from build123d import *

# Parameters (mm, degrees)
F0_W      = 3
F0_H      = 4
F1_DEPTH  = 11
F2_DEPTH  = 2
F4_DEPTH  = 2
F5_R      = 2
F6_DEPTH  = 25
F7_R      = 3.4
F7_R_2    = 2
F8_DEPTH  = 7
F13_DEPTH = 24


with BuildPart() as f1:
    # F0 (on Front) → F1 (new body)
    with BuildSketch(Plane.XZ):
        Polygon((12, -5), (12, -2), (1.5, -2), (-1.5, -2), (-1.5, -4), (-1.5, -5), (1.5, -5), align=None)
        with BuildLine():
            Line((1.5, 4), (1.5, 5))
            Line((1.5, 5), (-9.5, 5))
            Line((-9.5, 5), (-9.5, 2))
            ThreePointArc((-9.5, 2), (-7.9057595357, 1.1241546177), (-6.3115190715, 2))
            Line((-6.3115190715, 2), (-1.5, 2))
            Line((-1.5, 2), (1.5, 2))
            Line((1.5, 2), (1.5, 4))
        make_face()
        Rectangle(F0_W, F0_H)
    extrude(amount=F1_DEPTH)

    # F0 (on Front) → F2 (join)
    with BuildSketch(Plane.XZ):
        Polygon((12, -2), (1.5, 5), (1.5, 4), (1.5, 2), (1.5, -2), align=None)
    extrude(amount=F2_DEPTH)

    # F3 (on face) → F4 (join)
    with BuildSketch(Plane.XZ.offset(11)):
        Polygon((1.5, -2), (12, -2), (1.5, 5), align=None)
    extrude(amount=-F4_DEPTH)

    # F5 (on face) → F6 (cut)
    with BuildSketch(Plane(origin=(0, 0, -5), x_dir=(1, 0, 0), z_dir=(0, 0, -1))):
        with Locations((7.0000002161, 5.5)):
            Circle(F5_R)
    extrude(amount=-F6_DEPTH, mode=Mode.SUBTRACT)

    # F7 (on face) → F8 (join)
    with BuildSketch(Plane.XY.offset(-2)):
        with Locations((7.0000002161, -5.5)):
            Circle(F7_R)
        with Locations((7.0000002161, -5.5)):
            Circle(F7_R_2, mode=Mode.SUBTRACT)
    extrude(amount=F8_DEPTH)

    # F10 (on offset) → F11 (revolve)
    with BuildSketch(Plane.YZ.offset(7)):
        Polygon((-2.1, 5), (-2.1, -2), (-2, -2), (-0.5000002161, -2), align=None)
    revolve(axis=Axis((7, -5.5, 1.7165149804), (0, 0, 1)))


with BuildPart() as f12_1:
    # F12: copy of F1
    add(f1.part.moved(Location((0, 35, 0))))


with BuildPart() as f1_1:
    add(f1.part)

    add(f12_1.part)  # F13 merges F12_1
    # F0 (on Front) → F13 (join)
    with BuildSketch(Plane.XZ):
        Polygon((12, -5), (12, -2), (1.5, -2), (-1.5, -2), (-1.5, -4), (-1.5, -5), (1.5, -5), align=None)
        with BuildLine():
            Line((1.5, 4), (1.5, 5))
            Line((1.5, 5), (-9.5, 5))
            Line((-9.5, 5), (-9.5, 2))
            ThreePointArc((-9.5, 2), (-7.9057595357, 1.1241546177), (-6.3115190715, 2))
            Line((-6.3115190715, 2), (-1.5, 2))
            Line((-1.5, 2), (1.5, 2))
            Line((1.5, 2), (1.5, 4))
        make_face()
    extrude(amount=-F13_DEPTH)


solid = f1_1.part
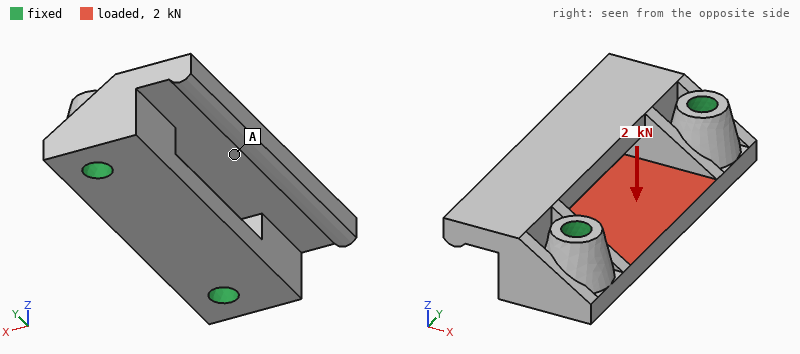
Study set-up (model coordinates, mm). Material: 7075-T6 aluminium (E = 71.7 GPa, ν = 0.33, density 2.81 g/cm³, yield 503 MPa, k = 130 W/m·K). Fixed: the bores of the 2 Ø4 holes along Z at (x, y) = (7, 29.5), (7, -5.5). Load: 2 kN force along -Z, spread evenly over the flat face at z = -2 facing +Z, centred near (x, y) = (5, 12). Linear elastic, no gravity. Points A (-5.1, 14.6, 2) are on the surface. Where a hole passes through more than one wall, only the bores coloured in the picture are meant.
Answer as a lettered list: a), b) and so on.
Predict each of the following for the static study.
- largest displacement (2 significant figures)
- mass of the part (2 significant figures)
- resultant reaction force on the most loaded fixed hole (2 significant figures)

a) 69 µm
b) 13 g
c) 1.0 kN
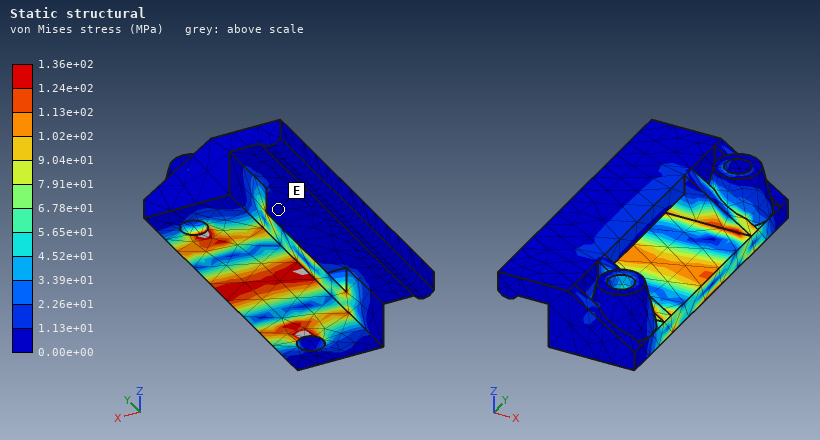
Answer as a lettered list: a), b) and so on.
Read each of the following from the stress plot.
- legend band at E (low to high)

a) 0.00e+00 to 1.13e+01 MPa
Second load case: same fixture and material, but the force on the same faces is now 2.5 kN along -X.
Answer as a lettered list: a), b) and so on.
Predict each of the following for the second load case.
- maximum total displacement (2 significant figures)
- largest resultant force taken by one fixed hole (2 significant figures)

a) 36 µm
b) 1.3 kN
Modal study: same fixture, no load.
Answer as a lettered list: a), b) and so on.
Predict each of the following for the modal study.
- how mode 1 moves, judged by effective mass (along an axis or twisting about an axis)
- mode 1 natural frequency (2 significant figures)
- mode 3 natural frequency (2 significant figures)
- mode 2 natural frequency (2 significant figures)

a) along Z
b) 10 kHz
c) 19 kHz
d) 17 kHz
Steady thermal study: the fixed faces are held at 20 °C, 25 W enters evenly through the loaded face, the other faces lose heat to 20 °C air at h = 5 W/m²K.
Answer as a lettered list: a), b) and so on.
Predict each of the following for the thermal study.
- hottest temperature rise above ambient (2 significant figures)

a) 23 K
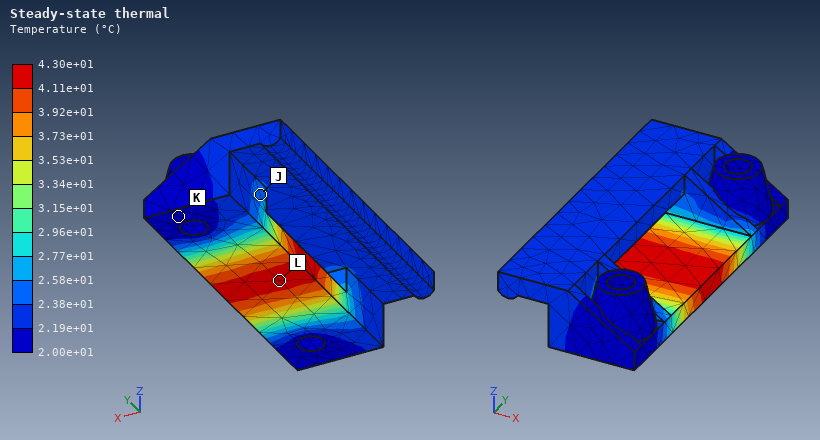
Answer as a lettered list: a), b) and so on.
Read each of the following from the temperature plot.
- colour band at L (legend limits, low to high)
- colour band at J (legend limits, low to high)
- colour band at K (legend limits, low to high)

a) 4.11e+01 to 4.30e+01 °C
b) 2.38e+01 to 2.58e+01 °C
c) 2.00e+01 to 2.19e+01 °C
